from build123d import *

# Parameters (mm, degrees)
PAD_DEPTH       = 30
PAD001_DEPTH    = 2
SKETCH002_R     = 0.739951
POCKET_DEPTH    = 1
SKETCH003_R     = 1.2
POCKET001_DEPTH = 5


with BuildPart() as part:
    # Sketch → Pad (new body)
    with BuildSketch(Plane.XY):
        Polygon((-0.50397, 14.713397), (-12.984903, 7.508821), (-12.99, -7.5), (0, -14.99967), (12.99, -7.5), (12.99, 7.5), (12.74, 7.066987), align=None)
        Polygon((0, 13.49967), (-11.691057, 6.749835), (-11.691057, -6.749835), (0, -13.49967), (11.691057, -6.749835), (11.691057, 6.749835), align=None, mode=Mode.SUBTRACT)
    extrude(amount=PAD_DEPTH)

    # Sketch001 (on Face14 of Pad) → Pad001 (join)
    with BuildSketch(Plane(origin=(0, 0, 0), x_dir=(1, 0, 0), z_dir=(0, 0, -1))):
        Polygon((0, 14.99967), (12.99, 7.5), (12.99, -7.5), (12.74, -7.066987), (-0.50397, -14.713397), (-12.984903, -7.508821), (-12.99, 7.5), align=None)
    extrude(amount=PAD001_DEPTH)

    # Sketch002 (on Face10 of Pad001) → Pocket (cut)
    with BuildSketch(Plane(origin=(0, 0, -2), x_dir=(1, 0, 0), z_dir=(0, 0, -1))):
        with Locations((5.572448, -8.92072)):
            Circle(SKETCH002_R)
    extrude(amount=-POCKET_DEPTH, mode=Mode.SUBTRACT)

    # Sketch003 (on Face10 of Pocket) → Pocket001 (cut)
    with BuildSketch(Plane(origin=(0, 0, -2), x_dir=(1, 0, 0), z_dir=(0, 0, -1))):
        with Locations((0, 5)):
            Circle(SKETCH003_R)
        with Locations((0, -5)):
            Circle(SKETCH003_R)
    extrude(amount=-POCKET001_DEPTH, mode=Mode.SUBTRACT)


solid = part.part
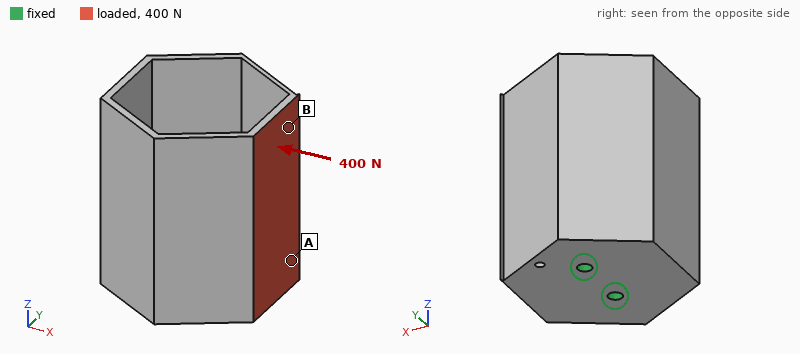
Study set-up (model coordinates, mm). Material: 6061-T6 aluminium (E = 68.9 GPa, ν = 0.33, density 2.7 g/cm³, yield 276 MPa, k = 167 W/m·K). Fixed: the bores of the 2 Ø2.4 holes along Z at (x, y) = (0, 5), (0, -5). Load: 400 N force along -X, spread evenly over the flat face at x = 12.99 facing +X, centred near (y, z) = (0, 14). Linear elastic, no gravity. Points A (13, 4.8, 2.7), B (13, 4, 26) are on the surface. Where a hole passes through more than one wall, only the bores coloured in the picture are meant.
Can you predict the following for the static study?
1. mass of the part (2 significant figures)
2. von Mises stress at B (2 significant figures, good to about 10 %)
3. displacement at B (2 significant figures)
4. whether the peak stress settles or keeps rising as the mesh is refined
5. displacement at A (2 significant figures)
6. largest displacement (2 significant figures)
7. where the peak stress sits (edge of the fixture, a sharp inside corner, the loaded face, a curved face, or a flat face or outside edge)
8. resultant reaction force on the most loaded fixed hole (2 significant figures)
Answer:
11 g
54 MPa
0.36 mm
keeps rising
0.15 mm
0.42 mm
edge of the fixture
200 N
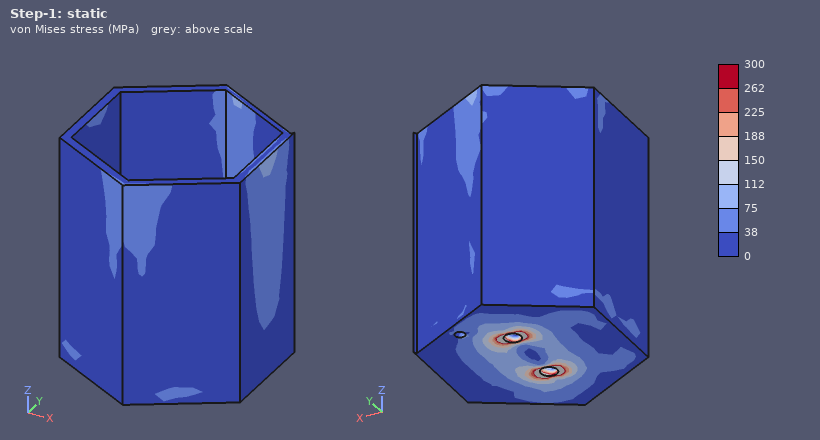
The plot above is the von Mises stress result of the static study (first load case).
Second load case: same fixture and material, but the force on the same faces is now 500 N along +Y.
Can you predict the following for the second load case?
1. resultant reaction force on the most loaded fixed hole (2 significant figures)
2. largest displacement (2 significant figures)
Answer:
780 N
0.22 mm
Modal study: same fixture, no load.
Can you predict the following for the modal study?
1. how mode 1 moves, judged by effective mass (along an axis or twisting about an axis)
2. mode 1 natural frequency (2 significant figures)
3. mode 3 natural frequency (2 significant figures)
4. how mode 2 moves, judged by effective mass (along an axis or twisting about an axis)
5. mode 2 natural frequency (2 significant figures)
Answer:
along X
2100 Hz
4900 Hz
along Y
3500 Hz
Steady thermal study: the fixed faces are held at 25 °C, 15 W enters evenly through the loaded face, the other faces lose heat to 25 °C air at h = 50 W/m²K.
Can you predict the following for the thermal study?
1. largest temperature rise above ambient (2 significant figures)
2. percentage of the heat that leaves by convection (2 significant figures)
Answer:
29 K
23 %
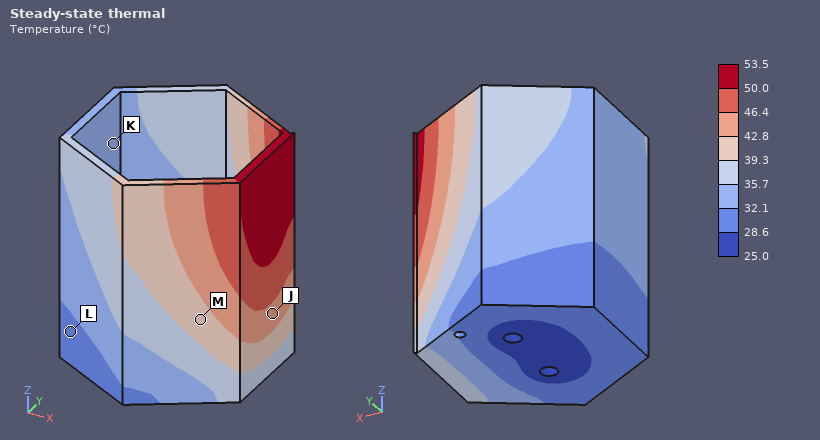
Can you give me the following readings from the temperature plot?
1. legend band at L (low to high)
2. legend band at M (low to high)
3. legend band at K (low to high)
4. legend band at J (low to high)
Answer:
28.6 to 32.1 °C
39.3 to 42.8 °C
32.1 to 35.7 °C
42.8 to 46.4 °C
